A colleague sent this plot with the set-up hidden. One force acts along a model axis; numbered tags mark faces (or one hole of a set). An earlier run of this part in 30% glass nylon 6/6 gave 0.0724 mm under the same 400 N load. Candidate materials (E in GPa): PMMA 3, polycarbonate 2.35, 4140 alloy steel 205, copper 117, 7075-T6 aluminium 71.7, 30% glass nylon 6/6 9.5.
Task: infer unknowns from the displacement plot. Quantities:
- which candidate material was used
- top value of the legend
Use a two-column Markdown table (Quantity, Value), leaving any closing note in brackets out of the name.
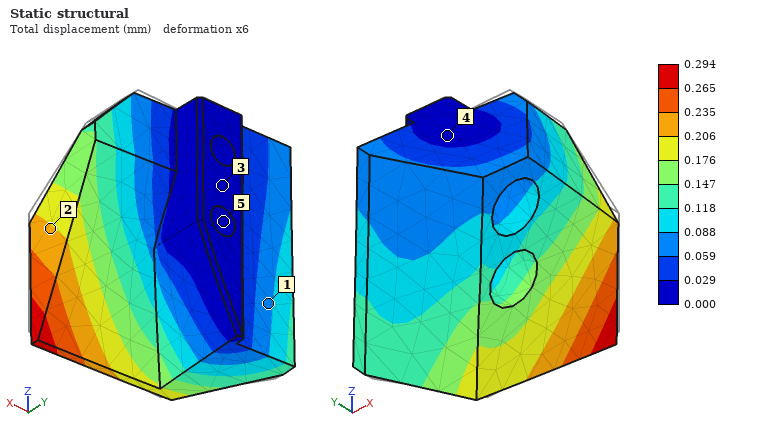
| Quantity | Value |
|---|---|
| which candidate material was used | polycarbonate |
| top value of the legend | 0.294 mm |
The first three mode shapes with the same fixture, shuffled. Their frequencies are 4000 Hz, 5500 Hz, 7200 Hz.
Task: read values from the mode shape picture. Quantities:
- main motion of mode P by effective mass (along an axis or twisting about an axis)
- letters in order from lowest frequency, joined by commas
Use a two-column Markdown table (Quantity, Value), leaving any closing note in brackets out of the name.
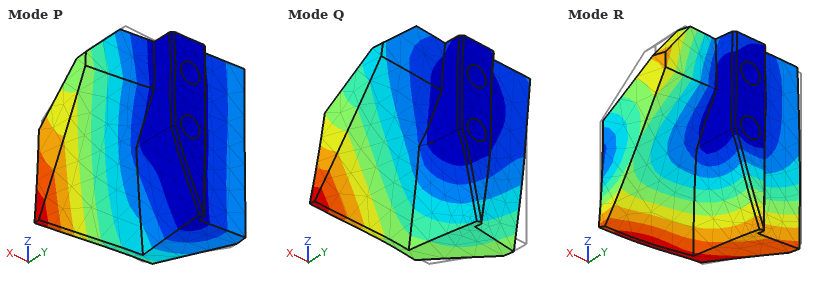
| Quantity | Value |
|---|---|
| main motion of mode P by effective mass | along X |
| letters in order from lowest frequency, joined by commas | P, Q, R |
